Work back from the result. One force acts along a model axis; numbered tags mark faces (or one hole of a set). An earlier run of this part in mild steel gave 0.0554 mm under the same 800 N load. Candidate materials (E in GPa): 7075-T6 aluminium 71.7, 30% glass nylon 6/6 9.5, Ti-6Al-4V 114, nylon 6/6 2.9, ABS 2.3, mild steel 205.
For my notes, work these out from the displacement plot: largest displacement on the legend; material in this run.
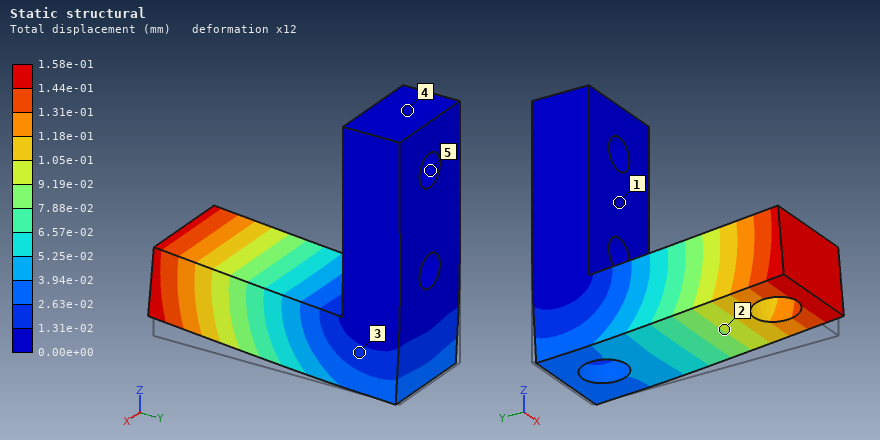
1.58e-01 mm
7075-T6 aluminium
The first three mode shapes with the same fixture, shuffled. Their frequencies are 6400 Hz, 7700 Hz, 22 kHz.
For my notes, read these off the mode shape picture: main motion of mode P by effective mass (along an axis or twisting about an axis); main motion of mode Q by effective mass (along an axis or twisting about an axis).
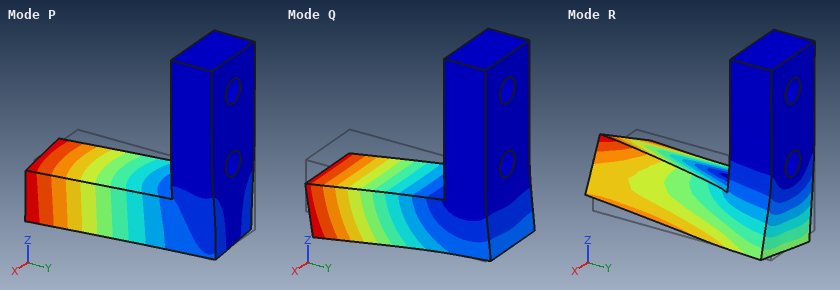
along X
along Z
